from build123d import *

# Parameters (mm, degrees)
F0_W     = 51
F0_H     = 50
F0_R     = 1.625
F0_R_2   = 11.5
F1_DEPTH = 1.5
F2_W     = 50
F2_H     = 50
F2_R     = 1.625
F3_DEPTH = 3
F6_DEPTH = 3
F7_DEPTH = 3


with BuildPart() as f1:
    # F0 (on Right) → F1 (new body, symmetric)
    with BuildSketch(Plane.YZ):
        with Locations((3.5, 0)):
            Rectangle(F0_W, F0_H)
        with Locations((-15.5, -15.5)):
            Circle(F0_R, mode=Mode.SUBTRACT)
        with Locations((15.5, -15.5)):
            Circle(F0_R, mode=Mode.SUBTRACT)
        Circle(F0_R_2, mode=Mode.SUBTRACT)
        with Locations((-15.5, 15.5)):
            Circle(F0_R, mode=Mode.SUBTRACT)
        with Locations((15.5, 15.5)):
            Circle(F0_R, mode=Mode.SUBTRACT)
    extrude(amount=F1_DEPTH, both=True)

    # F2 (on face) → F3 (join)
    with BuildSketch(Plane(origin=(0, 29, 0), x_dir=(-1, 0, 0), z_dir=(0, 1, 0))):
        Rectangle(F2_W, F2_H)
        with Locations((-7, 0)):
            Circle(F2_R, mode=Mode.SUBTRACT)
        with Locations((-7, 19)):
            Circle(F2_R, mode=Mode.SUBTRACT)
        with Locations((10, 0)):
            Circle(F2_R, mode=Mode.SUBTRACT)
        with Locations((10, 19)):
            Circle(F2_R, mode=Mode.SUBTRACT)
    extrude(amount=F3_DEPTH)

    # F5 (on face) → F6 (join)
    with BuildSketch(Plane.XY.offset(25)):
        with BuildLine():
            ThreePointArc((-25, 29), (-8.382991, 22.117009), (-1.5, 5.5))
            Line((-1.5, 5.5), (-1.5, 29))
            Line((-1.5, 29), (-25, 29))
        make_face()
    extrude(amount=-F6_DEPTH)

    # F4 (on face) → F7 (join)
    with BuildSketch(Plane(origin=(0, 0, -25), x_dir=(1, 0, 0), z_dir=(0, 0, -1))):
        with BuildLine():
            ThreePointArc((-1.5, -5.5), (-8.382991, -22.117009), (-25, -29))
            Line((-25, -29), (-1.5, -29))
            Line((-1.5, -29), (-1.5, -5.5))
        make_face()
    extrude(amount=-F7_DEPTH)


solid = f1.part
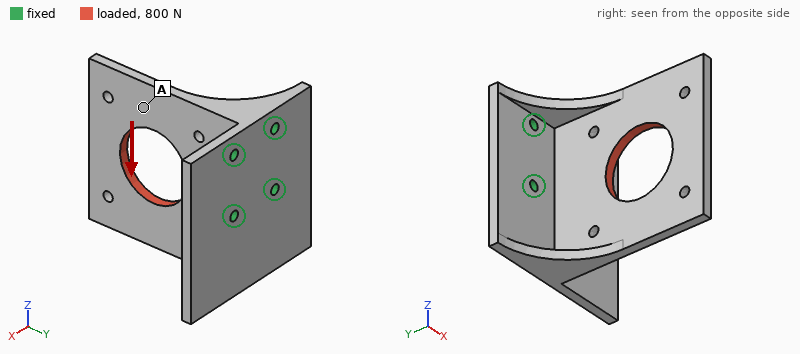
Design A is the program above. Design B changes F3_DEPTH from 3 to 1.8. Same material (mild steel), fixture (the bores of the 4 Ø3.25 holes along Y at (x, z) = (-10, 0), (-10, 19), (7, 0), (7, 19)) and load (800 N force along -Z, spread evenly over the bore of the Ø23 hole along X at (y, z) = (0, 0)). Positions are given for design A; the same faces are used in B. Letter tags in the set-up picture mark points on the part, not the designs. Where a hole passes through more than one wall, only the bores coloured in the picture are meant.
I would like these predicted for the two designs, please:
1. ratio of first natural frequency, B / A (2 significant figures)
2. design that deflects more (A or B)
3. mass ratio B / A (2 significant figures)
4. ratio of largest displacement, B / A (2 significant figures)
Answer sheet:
0.87
B
0.79
2.1
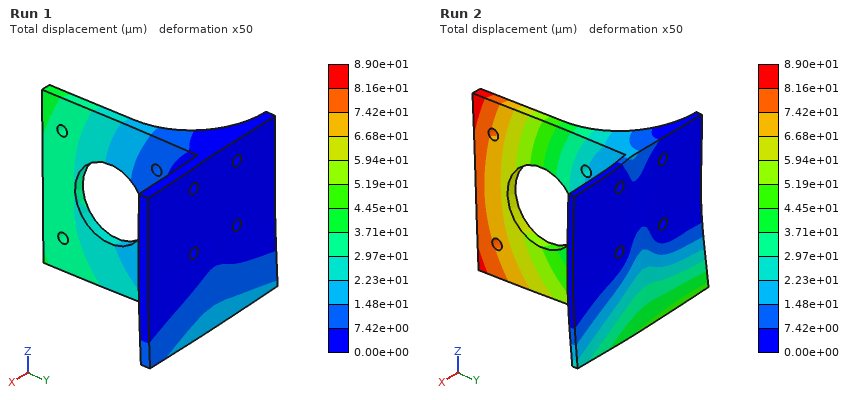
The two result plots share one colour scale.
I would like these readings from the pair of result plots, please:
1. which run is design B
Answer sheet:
Run 2
